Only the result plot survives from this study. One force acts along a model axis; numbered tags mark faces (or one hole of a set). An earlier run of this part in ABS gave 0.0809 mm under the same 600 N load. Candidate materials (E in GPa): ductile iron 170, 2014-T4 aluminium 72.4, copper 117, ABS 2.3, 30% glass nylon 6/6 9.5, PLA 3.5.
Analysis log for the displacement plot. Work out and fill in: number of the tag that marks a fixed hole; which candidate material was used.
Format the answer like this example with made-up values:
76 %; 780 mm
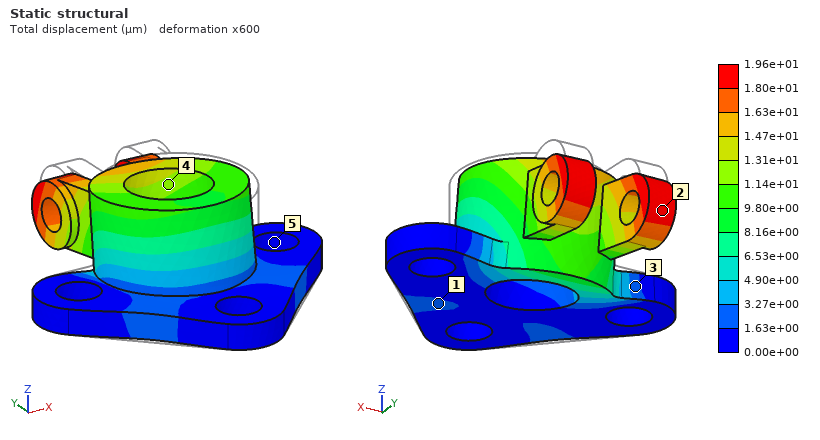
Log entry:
5; 30% glass nylon 6/6
